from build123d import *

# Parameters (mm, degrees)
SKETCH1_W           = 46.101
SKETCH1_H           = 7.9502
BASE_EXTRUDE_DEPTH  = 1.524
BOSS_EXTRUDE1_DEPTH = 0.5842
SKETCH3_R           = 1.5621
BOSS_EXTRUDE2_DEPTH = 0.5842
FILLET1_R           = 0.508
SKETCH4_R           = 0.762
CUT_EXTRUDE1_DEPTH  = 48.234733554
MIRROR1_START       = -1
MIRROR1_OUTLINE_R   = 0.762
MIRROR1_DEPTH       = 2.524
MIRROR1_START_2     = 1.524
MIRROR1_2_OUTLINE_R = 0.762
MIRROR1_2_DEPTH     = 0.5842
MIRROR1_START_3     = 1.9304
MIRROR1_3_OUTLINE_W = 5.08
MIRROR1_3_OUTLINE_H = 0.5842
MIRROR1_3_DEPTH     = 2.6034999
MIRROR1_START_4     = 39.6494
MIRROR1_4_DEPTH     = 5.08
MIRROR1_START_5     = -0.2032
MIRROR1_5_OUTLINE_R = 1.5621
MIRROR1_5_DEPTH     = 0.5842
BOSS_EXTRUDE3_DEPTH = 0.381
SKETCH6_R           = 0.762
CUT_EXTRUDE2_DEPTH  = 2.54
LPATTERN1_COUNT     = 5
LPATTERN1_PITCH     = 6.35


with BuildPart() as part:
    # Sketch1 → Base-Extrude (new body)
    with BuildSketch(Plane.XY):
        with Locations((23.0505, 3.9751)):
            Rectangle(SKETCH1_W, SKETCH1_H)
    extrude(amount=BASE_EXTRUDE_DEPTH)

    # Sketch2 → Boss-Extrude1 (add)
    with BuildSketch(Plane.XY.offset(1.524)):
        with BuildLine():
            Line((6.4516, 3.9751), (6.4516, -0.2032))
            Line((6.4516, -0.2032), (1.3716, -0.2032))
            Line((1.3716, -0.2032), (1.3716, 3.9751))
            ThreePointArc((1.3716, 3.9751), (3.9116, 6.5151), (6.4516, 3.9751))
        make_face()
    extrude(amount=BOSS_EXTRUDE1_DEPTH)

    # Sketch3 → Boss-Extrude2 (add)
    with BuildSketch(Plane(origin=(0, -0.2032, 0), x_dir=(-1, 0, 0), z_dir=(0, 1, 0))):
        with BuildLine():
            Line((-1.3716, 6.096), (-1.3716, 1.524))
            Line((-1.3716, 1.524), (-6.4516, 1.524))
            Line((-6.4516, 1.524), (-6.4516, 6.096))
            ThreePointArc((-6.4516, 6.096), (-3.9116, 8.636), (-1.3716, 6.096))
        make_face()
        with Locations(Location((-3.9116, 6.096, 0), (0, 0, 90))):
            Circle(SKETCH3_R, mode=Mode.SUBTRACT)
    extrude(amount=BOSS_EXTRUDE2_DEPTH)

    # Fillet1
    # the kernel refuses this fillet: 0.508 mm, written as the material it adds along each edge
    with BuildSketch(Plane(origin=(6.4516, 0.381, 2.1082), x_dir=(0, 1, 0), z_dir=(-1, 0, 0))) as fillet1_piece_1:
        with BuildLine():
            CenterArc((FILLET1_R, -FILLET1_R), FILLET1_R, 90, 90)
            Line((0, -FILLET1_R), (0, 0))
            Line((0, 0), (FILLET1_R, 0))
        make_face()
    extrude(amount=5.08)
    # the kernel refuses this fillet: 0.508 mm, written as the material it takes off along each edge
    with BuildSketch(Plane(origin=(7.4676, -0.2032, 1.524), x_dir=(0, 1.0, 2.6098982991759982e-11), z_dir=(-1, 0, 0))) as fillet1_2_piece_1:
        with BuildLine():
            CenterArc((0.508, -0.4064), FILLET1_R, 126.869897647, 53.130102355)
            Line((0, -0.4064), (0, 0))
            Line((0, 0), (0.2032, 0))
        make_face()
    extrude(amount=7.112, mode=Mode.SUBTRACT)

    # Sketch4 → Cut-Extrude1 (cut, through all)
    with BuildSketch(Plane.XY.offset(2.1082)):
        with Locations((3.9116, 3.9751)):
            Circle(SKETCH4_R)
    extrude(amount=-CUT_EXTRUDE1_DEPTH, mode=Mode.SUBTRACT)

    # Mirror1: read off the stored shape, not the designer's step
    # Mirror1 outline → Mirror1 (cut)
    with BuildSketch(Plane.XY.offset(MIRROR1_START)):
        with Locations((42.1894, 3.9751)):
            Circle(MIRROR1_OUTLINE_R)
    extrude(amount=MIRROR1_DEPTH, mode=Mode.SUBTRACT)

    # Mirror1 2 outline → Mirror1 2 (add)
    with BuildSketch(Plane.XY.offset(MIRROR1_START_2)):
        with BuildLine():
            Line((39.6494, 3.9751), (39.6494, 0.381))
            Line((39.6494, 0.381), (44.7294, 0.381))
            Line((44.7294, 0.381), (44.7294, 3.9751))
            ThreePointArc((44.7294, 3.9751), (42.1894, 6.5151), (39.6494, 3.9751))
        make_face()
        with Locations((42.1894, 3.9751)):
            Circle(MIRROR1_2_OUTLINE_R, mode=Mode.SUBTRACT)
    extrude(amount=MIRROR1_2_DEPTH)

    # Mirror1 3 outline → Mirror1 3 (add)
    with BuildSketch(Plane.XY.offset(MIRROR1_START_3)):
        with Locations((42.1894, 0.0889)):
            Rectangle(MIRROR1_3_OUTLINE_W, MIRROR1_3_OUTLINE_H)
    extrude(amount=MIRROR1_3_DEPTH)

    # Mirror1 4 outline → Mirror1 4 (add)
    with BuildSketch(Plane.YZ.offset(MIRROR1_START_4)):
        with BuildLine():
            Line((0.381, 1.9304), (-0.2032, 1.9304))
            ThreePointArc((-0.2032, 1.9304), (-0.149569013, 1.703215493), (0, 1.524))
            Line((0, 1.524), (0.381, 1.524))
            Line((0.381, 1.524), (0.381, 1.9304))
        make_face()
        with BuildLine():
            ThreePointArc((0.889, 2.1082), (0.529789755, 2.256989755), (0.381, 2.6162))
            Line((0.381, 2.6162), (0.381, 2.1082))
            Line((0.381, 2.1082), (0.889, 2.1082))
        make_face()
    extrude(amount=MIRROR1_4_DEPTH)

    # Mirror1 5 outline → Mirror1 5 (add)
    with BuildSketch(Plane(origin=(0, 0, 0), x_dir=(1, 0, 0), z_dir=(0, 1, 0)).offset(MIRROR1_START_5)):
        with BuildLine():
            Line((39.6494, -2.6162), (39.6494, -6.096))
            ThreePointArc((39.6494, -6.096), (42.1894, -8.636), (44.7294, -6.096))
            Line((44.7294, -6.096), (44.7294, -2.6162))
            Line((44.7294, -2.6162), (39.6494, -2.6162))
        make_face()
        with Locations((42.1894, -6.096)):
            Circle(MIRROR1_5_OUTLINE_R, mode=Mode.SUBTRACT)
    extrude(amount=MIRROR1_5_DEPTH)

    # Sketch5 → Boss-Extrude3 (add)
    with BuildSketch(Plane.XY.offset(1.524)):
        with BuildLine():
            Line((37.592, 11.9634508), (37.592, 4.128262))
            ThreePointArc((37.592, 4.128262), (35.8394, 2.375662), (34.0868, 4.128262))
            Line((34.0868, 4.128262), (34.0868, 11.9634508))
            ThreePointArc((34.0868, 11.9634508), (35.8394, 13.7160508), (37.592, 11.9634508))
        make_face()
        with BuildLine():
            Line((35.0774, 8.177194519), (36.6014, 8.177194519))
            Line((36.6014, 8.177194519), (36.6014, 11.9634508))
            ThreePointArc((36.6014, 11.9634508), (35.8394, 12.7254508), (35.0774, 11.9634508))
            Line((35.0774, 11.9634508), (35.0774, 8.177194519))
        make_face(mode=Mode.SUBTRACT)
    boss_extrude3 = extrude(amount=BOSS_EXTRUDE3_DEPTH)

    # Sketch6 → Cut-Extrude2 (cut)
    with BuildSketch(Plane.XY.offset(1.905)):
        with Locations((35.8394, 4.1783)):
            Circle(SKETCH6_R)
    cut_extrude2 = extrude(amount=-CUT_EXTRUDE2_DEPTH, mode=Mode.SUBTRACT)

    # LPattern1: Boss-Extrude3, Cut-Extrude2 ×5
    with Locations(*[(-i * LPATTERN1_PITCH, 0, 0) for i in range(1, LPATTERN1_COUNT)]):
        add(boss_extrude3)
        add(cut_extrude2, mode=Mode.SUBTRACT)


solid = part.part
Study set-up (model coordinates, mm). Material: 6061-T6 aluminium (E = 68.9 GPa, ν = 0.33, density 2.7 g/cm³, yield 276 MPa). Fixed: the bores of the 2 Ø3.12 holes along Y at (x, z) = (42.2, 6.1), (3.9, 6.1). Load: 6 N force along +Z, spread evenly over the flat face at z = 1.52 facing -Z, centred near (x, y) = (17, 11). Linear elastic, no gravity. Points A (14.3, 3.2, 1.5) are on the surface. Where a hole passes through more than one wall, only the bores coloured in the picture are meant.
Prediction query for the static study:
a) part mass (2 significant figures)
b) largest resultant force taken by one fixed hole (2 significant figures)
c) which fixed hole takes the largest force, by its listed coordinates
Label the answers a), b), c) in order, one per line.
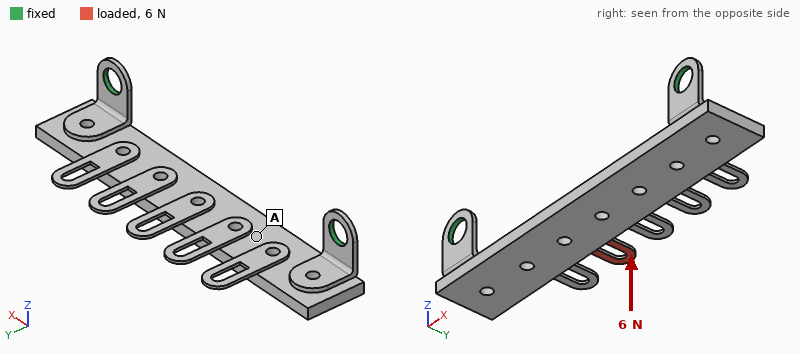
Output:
a) 1.8 g
b) 5.5 N
c) (3.9, 6.1)
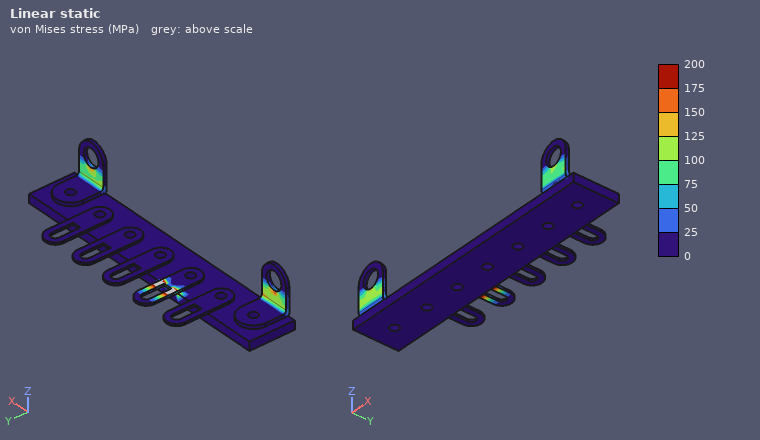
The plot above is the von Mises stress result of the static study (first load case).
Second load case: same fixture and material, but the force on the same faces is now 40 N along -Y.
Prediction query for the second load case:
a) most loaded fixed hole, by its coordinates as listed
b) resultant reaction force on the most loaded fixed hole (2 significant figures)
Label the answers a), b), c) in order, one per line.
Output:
a) (3.9, 6.1)
b) 29 N
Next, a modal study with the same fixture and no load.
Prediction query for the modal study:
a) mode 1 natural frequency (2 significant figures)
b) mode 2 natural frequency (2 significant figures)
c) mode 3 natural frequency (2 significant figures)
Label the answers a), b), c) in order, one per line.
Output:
a) 1400 Hz
b) 5300 Hz
c) 6000 Hz
